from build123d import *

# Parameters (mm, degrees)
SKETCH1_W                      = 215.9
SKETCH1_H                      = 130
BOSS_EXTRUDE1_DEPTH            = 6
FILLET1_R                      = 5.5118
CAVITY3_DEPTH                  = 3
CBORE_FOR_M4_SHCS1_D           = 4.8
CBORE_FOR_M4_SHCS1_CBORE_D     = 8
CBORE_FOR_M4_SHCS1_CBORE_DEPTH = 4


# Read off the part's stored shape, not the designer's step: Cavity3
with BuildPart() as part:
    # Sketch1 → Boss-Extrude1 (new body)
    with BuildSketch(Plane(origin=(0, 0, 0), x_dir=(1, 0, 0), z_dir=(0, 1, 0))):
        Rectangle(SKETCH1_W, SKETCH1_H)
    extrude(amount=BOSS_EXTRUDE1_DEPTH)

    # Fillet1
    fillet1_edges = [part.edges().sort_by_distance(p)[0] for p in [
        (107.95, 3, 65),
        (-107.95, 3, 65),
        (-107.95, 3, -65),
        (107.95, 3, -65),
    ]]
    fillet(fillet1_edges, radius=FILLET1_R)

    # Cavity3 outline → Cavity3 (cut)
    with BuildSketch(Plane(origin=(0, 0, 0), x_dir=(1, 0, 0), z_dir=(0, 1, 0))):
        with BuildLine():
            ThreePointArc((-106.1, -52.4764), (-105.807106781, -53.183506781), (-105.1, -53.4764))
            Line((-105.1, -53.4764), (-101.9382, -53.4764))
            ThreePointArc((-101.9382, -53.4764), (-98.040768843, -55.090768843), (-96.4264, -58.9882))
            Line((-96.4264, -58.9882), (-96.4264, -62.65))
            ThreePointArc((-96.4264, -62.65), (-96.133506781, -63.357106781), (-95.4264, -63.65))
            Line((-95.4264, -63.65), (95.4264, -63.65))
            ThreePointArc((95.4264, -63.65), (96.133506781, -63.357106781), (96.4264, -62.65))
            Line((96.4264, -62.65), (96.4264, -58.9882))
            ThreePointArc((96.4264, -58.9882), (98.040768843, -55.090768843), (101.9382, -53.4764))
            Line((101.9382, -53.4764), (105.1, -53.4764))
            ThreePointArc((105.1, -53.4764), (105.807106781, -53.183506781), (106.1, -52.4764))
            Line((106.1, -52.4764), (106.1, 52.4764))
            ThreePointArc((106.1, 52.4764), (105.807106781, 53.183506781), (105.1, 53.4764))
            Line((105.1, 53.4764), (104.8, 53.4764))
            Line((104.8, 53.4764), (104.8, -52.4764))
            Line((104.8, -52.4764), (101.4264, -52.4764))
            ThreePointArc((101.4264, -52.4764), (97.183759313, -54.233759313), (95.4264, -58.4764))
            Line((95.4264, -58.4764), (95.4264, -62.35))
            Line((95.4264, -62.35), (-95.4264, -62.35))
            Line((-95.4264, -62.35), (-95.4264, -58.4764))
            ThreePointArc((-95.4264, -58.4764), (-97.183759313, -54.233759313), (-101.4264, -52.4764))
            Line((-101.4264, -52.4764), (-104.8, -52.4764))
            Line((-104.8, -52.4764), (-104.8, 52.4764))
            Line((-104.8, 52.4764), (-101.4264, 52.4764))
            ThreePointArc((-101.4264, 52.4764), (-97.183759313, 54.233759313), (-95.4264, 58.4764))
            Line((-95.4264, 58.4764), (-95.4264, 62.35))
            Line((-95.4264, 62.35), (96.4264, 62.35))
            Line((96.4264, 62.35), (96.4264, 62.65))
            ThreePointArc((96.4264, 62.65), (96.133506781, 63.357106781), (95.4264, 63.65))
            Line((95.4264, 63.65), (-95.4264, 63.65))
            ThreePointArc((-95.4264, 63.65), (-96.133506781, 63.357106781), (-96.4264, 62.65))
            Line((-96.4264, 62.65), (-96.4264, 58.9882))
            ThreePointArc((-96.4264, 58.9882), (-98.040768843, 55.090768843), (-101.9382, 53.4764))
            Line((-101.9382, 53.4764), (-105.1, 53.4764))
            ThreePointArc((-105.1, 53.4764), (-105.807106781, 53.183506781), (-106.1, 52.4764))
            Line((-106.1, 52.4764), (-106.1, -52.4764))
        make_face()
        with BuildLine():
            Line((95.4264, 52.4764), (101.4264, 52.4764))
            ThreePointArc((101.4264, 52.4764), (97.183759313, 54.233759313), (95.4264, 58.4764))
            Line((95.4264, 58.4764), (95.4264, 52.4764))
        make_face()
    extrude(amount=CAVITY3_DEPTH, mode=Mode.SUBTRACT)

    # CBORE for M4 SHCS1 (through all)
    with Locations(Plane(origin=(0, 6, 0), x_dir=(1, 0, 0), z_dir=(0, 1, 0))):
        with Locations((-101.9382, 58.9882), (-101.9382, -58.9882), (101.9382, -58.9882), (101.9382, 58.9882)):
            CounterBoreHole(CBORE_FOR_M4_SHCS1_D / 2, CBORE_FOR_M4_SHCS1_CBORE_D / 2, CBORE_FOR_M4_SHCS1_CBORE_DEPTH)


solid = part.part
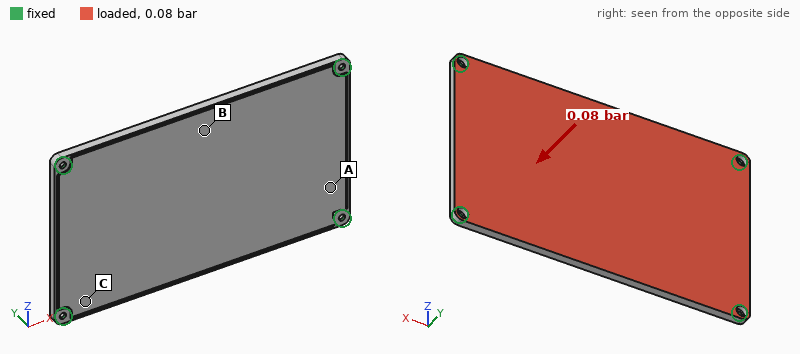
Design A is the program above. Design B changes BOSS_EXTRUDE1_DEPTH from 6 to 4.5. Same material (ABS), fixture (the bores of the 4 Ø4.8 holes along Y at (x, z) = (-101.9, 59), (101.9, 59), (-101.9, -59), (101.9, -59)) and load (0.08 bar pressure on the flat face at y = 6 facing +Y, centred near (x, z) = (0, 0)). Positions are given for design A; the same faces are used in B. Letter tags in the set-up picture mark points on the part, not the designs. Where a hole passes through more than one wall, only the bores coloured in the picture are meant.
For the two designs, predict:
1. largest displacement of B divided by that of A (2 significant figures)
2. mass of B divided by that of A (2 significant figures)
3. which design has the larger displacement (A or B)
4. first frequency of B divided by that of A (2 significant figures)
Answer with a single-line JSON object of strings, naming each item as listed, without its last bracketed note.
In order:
{"largest displacement of B divided by that of A": "2.2", "mass of B divided by that of A": "0.75", "which design has the larger displacement": "B", "first frequency of B divided by that of A": "0.78"}
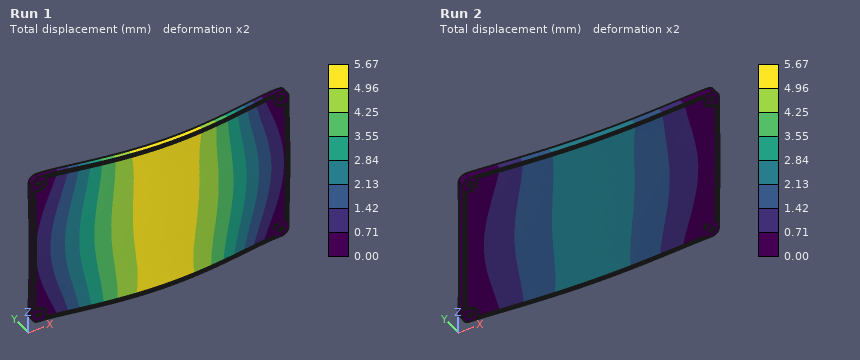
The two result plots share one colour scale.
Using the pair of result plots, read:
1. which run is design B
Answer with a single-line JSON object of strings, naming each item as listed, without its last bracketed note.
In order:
{"which run is design B": "Run 1"}
